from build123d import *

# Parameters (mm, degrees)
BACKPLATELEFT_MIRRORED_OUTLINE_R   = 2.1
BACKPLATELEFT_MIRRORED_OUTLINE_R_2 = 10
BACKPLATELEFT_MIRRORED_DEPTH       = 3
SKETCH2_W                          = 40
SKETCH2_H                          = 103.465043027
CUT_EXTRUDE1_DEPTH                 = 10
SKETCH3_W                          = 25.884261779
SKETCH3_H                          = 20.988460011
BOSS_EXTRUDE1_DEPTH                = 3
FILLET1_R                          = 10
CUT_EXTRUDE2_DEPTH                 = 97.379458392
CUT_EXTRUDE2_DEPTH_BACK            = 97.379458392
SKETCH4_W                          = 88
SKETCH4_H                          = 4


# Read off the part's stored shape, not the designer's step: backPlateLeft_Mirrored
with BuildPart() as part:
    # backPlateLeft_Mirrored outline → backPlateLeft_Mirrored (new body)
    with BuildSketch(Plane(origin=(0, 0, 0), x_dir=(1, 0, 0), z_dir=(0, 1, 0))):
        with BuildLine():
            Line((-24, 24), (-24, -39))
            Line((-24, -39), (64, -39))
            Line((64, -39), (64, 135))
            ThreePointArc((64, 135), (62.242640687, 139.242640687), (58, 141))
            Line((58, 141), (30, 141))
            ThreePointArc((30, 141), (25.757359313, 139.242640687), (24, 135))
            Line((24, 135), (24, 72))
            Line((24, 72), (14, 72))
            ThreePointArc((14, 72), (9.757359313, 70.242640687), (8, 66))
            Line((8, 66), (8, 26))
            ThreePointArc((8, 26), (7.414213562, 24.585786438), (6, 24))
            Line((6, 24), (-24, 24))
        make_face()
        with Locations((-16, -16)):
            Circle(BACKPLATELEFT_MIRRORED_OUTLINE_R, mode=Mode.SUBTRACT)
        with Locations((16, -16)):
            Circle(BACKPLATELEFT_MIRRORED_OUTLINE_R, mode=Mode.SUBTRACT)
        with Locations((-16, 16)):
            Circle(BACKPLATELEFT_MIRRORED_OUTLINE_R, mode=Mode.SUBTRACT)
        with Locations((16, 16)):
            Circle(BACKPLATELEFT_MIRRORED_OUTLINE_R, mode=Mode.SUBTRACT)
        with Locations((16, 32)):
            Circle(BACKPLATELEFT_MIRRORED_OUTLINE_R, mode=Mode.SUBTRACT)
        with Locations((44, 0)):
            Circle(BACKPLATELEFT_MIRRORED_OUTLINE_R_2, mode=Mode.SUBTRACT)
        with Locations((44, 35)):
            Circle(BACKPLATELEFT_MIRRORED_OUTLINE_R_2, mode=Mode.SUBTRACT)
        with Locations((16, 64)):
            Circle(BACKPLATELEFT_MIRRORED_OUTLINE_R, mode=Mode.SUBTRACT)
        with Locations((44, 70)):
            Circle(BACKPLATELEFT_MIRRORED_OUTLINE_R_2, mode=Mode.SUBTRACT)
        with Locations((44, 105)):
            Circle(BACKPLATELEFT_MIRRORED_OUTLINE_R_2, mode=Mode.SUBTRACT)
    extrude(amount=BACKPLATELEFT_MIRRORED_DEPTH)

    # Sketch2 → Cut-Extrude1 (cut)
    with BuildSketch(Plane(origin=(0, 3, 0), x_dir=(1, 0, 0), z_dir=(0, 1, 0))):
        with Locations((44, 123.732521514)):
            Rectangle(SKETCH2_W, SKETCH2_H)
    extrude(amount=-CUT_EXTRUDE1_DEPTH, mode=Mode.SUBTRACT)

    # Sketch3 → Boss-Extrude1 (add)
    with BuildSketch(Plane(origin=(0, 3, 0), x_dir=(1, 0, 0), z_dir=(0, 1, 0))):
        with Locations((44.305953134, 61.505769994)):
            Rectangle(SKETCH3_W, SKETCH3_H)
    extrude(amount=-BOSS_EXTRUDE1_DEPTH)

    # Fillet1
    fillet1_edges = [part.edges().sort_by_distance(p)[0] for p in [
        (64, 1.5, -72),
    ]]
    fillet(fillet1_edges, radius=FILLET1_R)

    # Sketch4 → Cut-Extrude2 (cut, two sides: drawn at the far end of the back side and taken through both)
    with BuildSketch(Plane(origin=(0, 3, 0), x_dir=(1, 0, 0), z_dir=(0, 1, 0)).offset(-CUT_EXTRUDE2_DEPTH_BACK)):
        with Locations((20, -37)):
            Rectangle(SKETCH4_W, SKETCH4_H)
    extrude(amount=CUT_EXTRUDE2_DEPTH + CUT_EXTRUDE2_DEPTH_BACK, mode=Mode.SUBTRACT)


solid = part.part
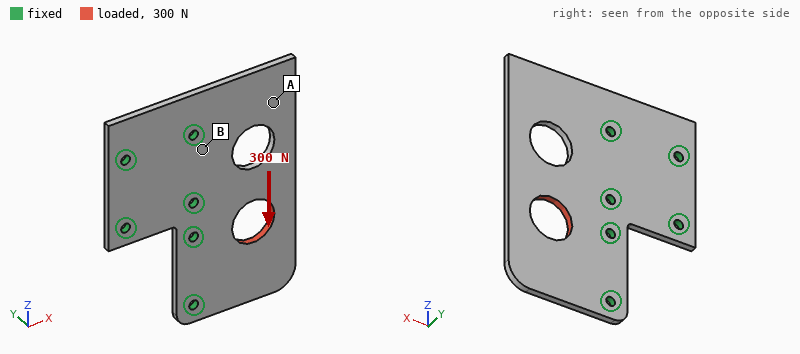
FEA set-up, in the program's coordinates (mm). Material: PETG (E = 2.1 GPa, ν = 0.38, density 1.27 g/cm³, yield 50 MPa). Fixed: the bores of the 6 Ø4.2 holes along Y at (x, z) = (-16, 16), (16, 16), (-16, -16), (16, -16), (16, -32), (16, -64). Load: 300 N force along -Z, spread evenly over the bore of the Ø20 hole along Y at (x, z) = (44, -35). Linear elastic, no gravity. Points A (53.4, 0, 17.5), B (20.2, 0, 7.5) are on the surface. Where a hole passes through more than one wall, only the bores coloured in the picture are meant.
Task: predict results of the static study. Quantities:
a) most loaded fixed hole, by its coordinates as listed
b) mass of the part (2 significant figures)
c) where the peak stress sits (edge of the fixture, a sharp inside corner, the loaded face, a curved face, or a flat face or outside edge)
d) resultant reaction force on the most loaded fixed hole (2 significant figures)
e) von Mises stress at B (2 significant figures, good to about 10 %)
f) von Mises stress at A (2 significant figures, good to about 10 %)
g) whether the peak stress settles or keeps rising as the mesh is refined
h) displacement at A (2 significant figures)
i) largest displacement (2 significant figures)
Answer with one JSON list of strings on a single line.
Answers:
["(16, -64)", "27 g", "edge of the fixture", "130 N", "1.8 MPa", "0.81 MPa", "keeps rising", "0.060 mm", "0.10 mm"]
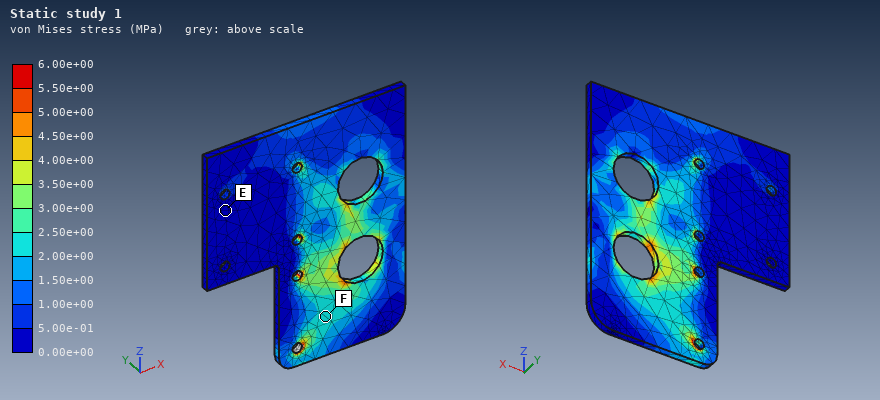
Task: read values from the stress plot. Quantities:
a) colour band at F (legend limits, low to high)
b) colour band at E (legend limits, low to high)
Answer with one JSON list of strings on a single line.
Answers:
["2.00e+00 to 2.50e+00 MPa", "0.00e+00 to 5.00e-01 MPa"]
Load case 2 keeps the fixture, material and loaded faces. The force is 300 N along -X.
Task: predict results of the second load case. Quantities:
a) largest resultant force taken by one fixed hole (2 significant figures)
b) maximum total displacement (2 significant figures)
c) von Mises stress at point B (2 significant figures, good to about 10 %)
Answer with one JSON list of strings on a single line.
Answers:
["110 N", "63 µm", "0.59 MPa"]
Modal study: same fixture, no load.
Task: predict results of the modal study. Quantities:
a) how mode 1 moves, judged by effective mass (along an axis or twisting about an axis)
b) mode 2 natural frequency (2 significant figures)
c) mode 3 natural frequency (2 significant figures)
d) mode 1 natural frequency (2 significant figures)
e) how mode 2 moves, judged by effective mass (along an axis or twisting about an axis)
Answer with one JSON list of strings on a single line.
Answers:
["along Y", "370 Hz", "660 Hz", "280 Hz", "twisting about X"]
